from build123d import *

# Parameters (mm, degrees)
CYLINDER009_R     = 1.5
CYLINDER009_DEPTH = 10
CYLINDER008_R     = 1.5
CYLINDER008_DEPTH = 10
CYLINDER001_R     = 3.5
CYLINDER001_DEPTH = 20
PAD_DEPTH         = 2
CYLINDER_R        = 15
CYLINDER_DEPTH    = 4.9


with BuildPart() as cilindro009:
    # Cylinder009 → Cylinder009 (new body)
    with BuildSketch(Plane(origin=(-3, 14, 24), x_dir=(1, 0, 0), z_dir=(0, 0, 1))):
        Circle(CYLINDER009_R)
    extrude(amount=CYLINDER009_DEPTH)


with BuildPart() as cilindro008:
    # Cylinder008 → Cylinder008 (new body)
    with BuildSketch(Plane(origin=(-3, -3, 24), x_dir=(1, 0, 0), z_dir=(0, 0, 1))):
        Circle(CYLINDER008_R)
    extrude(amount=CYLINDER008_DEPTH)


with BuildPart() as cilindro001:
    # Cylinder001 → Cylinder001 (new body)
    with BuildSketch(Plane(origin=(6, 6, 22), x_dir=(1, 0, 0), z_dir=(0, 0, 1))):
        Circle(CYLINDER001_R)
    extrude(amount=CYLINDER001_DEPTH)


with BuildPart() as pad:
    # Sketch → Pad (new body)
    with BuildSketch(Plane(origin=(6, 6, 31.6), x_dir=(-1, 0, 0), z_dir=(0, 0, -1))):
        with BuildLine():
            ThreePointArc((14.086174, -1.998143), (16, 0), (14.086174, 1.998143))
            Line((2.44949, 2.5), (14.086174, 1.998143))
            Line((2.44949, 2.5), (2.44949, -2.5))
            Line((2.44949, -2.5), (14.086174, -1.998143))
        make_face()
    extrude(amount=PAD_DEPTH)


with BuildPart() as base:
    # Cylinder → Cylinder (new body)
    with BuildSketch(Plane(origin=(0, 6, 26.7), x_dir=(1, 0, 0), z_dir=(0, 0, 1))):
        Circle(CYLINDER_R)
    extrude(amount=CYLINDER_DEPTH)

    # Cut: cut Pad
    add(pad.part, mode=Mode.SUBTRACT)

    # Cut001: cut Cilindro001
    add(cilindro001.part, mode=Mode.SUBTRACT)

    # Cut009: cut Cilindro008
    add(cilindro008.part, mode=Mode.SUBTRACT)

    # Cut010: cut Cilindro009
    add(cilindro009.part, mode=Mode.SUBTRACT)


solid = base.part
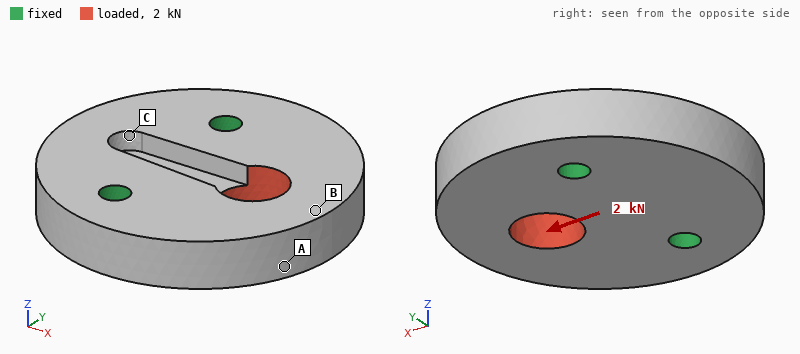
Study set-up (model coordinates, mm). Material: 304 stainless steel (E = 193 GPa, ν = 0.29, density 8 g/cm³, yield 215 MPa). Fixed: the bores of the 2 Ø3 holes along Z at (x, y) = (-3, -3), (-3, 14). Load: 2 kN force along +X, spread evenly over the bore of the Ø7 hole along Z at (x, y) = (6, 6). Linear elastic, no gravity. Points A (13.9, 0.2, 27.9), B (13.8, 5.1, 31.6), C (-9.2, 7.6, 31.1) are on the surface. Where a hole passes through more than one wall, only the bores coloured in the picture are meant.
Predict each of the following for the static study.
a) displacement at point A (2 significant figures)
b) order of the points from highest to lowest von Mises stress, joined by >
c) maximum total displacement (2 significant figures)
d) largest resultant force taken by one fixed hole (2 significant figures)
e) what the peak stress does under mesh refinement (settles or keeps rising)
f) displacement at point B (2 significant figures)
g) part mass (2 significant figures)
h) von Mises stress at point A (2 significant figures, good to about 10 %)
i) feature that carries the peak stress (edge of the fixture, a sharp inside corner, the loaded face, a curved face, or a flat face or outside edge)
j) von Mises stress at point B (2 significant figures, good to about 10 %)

1.6 µm
B > A > C
2.5 µm
1.1 kN
keeps rising
2.1 µm
25 g
13 MPa
edge of the fixture
21 MPa
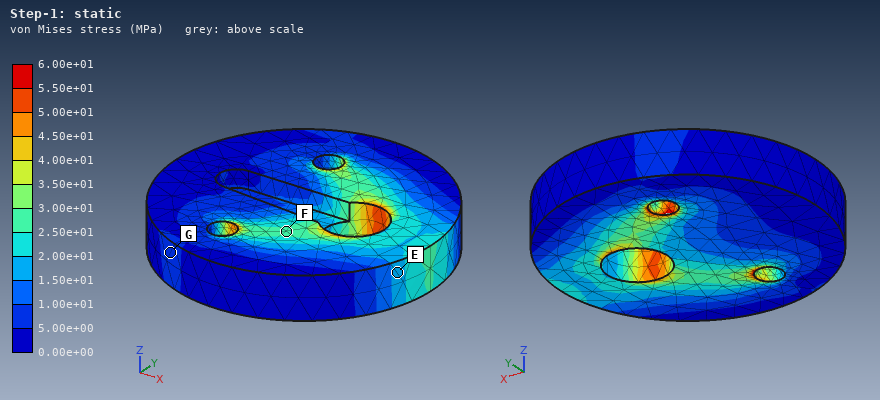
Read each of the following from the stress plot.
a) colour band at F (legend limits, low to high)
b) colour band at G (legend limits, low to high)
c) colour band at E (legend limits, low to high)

2.50e+01 to 3.00e+01 MPa
5.00e+00 to 1.00e+01 MPa
1.50e+01 to 2.00e+01 MPa
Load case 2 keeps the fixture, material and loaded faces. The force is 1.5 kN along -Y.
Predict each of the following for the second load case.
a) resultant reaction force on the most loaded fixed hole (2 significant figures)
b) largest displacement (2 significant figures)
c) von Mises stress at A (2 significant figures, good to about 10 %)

1.0 kN
4.2 µm
15 MPa
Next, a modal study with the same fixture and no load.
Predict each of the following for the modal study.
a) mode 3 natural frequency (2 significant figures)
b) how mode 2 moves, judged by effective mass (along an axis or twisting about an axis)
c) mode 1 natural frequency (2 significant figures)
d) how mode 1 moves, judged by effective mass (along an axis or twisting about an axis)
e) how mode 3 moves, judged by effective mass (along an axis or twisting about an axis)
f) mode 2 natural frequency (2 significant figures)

27 kHz
twisting about X
13 kHz
along Z
along Z
26 kHz
